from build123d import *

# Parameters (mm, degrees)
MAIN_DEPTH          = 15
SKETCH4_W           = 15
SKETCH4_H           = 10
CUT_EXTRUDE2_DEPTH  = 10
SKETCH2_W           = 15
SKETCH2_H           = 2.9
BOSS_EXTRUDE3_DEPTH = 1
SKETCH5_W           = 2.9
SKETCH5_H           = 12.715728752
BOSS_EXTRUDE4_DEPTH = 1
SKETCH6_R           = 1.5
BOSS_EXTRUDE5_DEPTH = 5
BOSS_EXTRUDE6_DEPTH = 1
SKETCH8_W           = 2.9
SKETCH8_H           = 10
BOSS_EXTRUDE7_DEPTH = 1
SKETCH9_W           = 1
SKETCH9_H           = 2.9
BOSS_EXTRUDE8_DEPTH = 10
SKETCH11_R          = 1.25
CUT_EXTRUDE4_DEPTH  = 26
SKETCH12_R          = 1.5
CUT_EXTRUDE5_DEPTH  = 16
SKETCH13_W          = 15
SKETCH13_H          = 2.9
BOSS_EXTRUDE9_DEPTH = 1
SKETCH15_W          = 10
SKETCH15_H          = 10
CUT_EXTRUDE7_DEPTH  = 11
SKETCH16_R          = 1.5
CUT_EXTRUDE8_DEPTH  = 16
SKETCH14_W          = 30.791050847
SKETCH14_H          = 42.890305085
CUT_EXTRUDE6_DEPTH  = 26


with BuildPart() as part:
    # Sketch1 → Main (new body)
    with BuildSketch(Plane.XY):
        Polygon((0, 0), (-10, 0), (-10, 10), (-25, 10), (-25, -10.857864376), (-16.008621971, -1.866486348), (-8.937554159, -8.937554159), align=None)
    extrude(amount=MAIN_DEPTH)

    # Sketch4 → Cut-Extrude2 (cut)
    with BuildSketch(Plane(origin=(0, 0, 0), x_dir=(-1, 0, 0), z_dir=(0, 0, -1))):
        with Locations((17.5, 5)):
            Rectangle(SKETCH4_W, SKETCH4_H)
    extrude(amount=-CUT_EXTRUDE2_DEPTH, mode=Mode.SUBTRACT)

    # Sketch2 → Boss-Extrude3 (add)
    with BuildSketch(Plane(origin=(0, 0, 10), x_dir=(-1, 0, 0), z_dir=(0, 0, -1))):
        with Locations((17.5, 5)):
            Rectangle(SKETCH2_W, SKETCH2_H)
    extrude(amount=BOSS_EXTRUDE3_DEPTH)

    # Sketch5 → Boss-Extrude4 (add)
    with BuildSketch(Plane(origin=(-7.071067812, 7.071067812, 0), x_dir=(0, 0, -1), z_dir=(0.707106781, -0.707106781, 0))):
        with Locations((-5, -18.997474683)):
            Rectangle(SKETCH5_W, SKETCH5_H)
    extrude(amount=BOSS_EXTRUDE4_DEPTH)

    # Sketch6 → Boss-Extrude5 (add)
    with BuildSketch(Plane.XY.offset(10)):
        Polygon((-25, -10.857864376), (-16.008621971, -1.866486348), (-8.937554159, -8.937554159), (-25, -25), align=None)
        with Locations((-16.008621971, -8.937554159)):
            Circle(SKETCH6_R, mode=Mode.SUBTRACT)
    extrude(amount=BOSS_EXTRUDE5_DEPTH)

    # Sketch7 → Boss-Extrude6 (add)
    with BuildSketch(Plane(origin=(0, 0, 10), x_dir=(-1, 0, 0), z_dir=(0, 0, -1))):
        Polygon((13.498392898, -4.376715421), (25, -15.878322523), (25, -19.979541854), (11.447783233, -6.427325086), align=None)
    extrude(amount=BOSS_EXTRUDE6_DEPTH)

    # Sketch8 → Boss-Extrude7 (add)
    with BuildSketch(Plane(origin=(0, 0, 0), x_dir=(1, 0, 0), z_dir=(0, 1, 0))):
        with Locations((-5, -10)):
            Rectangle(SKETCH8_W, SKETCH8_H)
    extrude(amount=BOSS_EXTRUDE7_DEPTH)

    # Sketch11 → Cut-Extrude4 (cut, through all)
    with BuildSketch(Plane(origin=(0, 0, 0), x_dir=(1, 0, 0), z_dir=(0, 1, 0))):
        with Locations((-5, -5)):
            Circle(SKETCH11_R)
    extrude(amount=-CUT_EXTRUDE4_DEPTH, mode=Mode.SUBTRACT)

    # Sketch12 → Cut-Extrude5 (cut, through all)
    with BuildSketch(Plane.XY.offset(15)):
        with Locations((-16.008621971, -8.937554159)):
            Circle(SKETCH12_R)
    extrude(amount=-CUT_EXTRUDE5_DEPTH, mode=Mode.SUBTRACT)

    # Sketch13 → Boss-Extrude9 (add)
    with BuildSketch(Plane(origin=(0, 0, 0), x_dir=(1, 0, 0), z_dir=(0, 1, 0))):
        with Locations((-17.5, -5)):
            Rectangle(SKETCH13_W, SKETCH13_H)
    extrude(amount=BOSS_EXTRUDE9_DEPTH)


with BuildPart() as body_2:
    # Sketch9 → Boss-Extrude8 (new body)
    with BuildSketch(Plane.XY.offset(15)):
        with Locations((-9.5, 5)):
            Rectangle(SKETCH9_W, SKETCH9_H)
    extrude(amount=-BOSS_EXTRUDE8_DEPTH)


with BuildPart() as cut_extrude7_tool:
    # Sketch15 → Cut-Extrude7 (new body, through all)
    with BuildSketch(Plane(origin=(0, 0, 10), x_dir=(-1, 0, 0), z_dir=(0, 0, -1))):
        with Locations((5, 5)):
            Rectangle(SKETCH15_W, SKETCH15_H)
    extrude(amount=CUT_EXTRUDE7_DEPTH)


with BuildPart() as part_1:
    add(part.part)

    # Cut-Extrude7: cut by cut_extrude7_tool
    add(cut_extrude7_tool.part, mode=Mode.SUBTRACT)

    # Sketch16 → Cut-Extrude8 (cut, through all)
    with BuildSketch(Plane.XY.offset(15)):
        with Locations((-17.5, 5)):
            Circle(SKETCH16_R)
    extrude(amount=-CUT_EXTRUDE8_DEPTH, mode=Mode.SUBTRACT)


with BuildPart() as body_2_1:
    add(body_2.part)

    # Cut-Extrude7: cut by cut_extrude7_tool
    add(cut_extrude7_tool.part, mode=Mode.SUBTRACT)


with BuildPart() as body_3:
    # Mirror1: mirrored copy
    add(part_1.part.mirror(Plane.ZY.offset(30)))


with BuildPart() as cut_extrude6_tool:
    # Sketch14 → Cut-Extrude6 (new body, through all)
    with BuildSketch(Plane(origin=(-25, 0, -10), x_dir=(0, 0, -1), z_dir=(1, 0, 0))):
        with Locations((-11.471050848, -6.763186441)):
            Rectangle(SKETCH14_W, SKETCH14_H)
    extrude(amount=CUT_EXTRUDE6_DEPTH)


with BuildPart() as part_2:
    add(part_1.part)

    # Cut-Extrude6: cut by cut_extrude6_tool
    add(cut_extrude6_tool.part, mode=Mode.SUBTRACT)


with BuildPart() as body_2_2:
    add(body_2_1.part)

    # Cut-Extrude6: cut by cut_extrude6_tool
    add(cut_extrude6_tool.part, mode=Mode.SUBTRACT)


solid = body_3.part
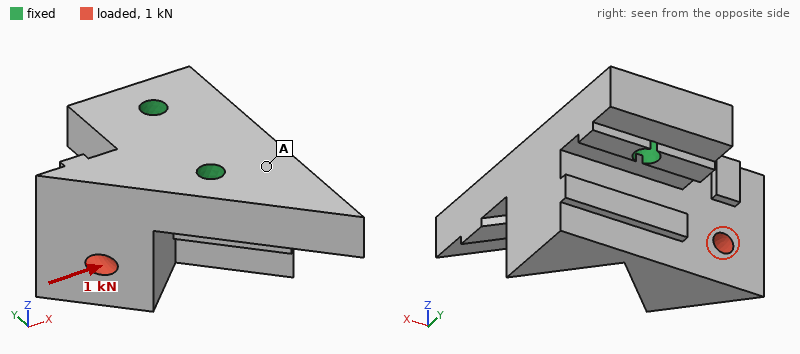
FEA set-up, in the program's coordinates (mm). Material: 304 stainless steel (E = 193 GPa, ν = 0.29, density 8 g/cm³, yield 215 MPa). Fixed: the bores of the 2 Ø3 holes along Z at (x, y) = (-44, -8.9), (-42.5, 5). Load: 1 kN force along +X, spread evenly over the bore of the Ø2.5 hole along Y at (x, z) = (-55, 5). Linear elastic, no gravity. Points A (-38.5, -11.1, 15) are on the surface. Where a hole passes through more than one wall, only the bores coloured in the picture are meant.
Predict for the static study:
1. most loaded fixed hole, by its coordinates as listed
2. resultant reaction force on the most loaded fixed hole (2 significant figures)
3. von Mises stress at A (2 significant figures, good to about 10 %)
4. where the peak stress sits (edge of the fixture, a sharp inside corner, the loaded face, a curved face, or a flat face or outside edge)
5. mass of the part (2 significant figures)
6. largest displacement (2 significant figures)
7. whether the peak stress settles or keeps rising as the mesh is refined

(-44, -8.9)
570 N
12 MPa
edge of the fixture
30 g
12 µm
keeps rising
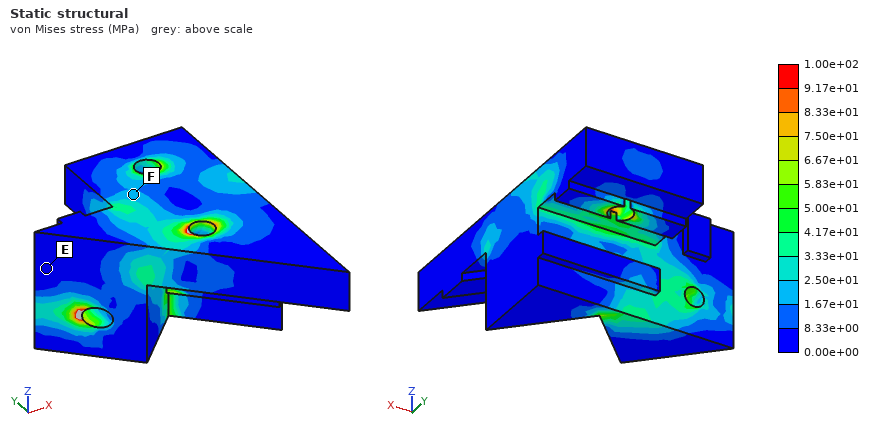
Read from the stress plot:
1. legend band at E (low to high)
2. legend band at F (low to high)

0.00e+00 to 8.33e+00 MPa
1.67e+01 to 2.50e+01 MPa
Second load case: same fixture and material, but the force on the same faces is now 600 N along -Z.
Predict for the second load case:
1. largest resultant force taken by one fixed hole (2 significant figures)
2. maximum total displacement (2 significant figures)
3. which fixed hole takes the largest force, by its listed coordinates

410 N
12 µm
(-44, -8.9)
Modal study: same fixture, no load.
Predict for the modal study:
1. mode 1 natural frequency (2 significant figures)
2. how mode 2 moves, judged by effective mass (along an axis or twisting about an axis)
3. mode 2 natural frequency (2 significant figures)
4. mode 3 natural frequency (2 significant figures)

15 kHz
along Y
22 kHz
24 kHz
